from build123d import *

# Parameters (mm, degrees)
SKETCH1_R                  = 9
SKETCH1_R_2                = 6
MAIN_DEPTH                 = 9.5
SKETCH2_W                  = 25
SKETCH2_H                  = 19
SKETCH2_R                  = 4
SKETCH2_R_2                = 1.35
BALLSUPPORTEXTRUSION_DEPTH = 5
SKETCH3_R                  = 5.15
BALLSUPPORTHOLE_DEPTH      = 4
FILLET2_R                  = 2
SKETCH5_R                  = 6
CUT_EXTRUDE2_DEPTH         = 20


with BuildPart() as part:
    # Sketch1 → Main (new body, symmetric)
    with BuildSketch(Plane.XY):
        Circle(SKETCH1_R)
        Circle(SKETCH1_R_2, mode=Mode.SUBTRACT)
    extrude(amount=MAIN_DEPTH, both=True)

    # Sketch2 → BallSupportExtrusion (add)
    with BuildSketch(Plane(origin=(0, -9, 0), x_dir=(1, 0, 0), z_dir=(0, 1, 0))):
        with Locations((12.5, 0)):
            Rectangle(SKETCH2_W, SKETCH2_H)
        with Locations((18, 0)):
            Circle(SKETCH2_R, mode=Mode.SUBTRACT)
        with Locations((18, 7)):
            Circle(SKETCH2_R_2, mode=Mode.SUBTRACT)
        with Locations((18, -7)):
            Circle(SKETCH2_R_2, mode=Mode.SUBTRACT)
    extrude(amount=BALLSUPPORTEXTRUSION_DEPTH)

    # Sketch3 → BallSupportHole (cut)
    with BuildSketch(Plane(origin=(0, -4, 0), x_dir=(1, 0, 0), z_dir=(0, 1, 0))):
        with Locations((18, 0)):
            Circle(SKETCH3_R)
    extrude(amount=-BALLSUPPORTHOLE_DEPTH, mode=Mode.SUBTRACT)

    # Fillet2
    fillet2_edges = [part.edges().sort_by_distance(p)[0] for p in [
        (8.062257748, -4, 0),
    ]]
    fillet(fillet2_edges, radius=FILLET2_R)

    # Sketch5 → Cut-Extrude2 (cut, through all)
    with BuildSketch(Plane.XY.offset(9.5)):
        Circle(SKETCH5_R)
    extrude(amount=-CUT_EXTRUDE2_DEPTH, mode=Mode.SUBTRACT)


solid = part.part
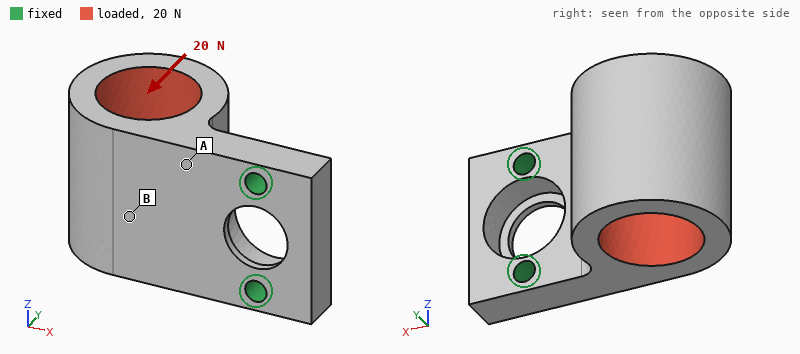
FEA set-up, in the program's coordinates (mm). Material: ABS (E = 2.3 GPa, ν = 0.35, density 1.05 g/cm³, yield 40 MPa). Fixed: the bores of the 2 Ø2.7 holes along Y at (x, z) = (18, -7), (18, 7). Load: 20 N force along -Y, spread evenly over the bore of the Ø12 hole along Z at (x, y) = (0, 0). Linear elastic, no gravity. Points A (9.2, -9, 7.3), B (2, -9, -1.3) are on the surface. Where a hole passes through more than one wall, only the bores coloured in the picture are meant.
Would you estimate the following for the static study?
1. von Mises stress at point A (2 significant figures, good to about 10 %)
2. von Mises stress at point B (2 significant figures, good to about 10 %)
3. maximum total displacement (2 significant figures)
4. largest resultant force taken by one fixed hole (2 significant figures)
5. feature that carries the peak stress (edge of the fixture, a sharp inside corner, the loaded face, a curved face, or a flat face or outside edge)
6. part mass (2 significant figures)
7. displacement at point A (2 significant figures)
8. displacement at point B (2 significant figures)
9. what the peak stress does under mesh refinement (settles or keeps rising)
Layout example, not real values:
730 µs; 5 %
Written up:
2.3 MPa; 1.0 MPa; 0.22 mm; 10 N; edge of the fixture; 4.3 g; 0.042 mm; 0.10 mm; keeps rising
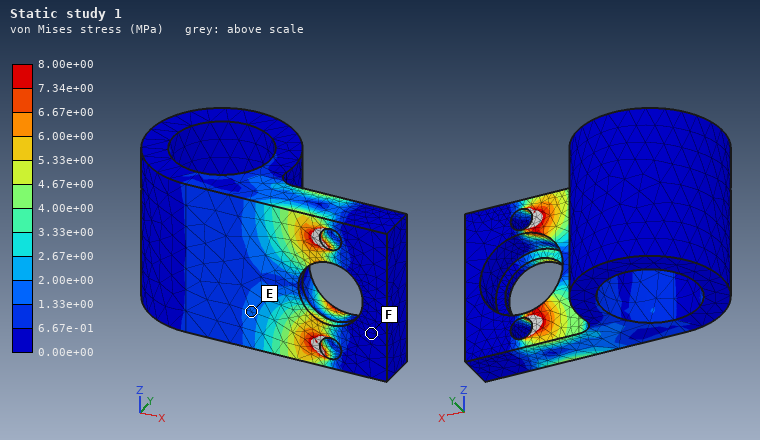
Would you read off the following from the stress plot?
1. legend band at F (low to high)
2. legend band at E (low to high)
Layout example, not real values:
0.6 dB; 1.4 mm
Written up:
0.00e+00 to 6.67e-01 MPa; 1.33e+00 to 2.00e+00 MPa
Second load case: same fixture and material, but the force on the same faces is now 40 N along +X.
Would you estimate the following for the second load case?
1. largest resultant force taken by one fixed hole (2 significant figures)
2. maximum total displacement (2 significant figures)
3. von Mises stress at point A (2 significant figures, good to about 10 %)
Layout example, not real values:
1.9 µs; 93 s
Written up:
21 N; 0.22 mm; 2.4 MPa
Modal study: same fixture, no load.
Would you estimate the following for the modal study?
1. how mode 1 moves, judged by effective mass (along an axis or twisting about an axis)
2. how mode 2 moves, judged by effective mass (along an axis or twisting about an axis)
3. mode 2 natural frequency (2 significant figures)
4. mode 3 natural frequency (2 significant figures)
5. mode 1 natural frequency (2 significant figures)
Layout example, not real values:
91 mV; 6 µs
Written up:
along Y; along Z; 2500 Hz; 4700 Hz; 960 Hz
